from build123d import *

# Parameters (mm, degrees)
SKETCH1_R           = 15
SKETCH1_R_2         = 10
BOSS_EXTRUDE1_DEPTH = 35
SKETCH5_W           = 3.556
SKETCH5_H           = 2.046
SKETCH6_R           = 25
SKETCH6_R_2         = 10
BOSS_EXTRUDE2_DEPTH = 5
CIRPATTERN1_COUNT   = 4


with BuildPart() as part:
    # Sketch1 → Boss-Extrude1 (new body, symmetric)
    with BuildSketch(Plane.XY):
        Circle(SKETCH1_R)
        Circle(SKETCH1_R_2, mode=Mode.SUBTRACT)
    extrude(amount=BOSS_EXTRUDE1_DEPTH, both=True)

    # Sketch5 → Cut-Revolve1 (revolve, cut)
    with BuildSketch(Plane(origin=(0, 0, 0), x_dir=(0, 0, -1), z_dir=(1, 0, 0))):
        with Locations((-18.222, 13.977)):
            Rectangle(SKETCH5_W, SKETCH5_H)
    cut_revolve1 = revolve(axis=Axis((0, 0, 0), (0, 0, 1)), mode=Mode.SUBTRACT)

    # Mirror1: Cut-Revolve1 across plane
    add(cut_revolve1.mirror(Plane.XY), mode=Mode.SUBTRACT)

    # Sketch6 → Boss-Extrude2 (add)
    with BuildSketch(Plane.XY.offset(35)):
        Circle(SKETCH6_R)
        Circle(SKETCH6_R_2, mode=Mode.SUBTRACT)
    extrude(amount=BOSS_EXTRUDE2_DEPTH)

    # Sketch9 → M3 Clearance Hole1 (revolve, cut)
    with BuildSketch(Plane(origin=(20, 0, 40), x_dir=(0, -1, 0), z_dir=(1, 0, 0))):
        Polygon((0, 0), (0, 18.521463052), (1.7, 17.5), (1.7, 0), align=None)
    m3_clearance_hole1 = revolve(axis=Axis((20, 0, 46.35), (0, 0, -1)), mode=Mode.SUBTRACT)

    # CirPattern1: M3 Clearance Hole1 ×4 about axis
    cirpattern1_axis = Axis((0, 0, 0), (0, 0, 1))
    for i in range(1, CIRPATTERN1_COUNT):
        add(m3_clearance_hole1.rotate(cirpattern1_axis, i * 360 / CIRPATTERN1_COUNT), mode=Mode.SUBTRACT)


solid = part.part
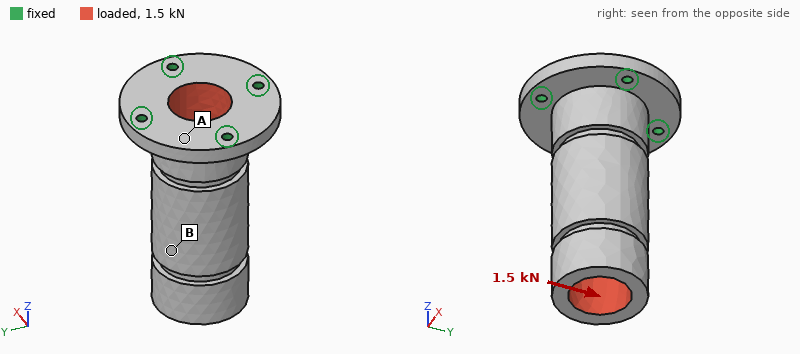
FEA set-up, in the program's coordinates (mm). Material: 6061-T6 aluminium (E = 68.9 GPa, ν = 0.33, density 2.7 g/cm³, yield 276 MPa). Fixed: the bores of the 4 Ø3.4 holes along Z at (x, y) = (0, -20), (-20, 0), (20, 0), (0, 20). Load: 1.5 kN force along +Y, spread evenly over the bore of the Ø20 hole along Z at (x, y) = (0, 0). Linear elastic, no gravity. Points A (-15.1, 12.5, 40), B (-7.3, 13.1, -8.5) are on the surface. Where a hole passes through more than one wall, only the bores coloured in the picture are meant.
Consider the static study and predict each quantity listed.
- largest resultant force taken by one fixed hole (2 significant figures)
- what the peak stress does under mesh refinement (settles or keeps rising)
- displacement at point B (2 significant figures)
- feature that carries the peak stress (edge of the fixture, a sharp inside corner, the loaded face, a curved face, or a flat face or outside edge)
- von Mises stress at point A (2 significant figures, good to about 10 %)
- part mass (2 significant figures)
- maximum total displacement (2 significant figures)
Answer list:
1.5 kN
keeps rising
58 µm
edge of the fixture
15 MPa
93 g
93 µm
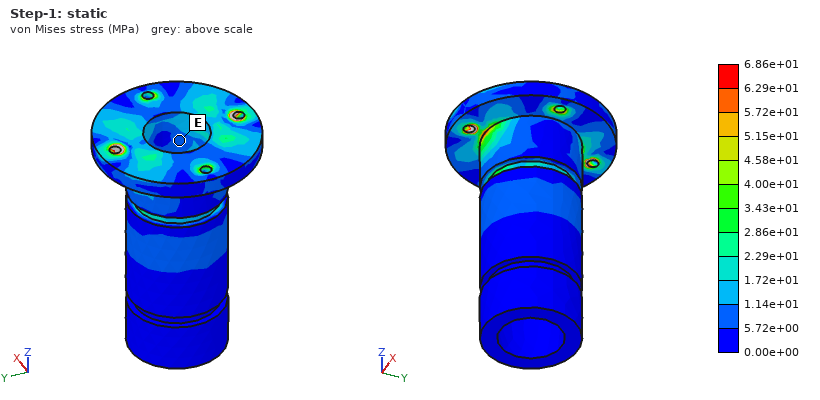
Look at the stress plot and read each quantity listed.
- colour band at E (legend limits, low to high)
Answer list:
5.72e+00 to 1.14e+01 MPa
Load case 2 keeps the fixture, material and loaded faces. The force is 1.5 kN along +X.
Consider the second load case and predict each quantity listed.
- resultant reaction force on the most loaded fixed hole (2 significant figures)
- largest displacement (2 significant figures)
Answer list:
1.5 kN
93 µm
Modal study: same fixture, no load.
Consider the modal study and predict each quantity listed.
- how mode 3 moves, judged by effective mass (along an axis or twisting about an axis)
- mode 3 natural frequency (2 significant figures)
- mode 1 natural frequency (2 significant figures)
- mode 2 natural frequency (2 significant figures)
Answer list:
twisting about Z
9900 Hz
2800 Hz
2800 Hz
